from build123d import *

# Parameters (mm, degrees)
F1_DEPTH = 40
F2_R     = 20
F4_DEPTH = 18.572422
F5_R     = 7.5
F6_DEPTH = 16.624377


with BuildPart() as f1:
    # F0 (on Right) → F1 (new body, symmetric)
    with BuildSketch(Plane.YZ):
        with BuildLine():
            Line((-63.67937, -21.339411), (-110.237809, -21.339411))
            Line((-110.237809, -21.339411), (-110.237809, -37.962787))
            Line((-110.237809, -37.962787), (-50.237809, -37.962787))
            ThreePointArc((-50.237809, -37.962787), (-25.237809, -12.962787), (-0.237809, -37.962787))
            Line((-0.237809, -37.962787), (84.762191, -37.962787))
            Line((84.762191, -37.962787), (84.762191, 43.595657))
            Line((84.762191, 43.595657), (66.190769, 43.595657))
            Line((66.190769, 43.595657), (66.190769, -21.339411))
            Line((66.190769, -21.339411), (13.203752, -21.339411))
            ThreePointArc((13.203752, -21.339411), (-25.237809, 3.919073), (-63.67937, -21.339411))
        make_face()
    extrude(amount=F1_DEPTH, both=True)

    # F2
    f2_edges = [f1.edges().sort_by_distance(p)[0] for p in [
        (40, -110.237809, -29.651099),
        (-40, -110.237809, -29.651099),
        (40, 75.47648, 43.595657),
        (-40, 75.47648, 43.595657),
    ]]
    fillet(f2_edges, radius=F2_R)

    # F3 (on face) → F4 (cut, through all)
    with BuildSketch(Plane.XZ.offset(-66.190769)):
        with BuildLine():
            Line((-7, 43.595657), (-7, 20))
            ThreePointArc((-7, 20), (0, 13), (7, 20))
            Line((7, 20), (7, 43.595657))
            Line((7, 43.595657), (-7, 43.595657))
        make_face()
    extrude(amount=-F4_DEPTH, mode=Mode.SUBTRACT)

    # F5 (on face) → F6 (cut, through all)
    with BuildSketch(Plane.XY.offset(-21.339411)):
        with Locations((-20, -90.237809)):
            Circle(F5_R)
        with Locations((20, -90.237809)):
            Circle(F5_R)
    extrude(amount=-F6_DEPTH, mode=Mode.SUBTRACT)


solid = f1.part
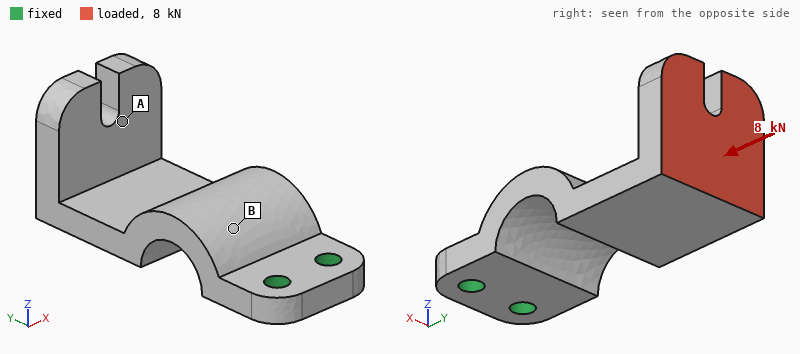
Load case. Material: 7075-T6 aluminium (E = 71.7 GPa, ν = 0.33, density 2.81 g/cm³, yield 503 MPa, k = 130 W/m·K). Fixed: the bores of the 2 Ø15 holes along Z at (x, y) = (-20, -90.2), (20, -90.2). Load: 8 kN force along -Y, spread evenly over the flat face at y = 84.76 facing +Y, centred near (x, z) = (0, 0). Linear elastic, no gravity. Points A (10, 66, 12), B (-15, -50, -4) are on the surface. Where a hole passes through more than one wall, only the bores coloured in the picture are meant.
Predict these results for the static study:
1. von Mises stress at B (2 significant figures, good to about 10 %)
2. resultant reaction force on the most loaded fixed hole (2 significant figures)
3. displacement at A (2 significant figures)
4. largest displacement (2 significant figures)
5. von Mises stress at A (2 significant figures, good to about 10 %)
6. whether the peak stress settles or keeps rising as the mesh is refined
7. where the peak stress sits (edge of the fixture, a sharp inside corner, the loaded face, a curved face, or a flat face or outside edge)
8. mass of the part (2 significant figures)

23 MPa
4.1 kN
1.0 mm
1.5 mm
12 MPa
keeps rising
edge of the fixture
1.0 kg
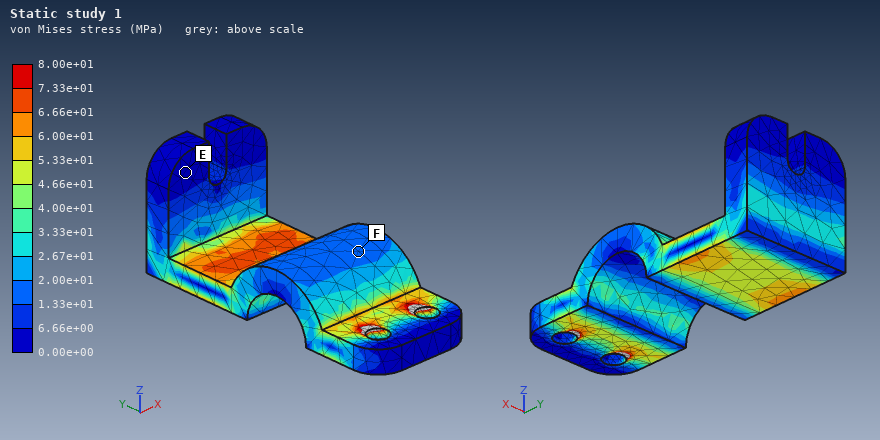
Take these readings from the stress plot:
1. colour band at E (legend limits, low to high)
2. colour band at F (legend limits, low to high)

0.00e+00 to 6.66e+00 MPa
1.33e+01 to 2.00e+01 MPa
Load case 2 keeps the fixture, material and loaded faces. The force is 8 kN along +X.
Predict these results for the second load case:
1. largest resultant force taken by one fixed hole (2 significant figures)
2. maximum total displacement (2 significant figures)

28 kN
1.2 mm
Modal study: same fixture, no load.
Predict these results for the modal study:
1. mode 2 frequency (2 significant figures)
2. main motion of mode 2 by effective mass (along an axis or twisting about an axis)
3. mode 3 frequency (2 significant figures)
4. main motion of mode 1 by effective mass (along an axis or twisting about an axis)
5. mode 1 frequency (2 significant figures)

760 Hz
along X
1100 Hz
along Z
280 Hz
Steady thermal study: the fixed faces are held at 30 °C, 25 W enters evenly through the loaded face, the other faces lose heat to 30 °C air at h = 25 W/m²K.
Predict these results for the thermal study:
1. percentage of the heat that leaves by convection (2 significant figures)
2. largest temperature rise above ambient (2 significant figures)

44 %
19 K
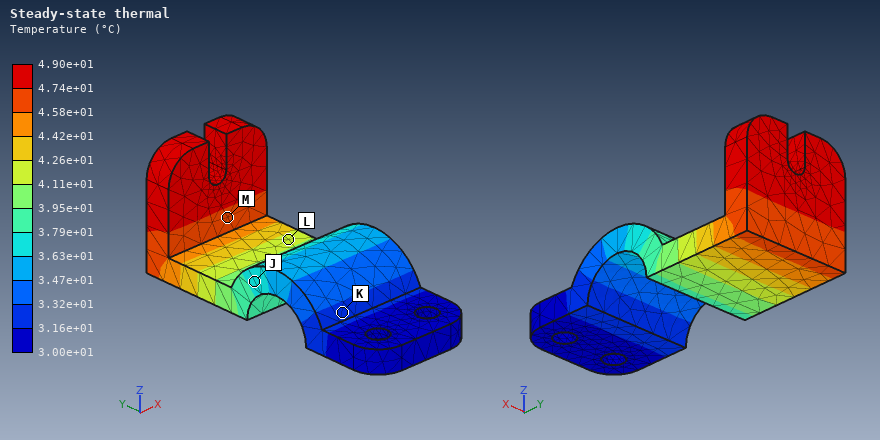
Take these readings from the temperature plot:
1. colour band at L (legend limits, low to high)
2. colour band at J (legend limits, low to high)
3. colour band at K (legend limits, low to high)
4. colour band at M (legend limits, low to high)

4.11e+01 to 4.26e+01 °C
3.63e+01 to 3.79e+01 °C
3.16e+01 to 3.32e+01 °C
4.58e+01 to 4.74e+01 °C
